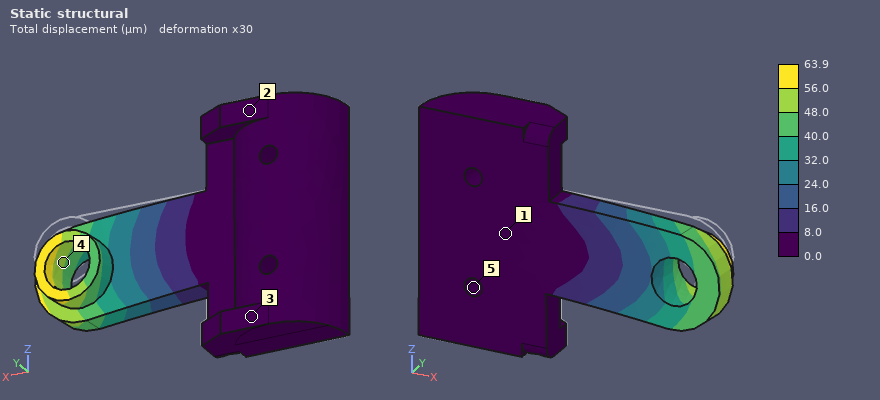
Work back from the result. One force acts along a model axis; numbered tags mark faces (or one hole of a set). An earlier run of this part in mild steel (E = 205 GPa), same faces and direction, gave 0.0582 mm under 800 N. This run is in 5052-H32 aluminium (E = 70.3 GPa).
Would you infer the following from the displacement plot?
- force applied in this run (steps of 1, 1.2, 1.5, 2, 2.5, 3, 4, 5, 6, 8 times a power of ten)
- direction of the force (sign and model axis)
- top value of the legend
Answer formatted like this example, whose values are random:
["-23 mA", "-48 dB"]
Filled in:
["300 N", "-Z", "63.9 µm"]
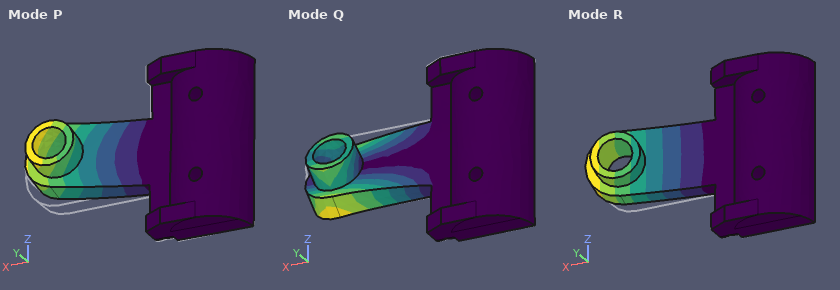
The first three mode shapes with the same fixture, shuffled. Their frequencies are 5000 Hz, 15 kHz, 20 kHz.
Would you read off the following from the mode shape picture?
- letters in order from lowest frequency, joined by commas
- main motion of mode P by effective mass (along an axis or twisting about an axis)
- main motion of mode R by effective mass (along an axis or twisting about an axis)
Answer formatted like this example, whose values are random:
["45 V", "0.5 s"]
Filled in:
["R, P, Q", "along Z", "along Y"]
